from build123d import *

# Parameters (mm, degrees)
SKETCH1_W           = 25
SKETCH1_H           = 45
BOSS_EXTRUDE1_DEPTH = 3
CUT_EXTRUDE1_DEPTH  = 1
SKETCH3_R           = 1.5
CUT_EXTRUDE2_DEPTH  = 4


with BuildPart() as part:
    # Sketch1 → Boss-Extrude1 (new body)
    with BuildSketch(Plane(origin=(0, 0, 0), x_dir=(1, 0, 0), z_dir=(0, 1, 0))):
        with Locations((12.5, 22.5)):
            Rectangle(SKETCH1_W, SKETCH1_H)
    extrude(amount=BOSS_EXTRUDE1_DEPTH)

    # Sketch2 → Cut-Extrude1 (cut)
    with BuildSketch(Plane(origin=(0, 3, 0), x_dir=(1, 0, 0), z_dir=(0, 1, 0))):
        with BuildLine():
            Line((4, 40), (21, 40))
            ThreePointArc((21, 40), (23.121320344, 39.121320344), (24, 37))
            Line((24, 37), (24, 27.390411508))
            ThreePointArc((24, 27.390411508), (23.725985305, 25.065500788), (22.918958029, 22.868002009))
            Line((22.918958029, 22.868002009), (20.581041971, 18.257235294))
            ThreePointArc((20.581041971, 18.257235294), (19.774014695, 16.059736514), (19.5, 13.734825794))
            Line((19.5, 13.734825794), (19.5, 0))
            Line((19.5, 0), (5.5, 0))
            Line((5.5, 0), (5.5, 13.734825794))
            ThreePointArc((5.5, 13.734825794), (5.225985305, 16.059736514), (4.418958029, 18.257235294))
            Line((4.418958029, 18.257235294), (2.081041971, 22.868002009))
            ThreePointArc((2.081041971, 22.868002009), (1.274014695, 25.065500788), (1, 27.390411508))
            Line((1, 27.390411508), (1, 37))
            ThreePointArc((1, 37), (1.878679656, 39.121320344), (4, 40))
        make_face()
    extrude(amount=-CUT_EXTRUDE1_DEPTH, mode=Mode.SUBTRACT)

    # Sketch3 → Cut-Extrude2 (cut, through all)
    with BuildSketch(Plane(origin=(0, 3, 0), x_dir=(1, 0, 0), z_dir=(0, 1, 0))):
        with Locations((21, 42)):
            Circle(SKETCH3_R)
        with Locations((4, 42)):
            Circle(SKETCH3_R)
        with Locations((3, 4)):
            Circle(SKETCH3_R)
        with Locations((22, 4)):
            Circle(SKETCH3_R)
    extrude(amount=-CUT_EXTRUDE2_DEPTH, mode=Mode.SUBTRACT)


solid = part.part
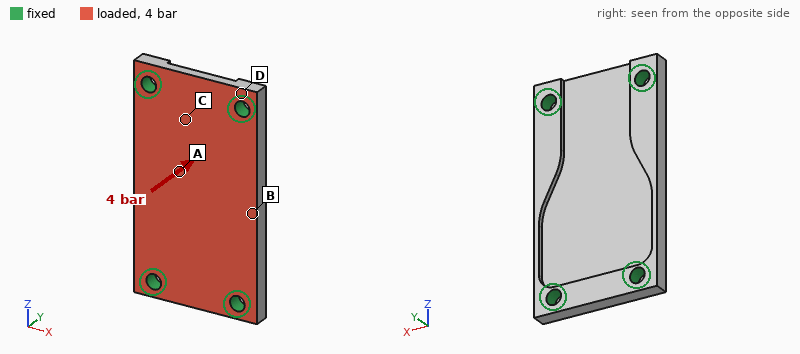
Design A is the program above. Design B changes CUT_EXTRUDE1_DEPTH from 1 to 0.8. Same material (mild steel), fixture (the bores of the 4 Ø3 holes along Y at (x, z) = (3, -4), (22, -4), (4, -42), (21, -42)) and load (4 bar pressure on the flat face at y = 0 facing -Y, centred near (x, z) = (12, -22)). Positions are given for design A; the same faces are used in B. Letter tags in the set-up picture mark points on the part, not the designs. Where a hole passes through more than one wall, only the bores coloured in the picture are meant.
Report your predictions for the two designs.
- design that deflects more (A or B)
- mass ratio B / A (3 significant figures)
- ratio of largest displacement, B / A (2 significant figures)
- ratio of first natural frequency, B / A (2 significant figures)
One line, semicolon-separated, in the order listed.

A; 1.06; 0.86; 1.0
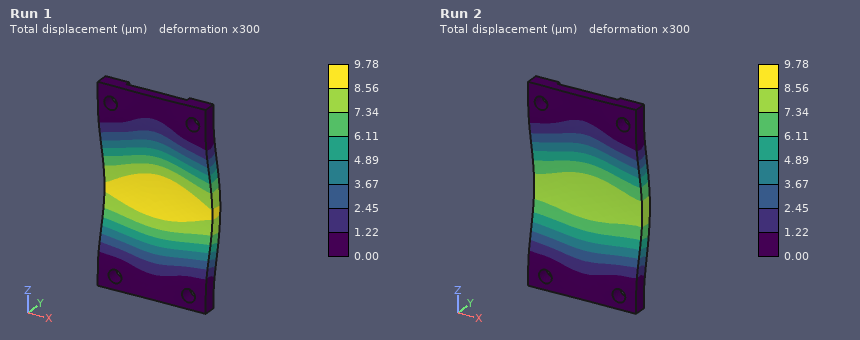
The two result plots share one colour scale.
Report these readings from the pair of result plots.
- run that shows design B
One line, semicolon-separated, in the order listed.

Run 2
